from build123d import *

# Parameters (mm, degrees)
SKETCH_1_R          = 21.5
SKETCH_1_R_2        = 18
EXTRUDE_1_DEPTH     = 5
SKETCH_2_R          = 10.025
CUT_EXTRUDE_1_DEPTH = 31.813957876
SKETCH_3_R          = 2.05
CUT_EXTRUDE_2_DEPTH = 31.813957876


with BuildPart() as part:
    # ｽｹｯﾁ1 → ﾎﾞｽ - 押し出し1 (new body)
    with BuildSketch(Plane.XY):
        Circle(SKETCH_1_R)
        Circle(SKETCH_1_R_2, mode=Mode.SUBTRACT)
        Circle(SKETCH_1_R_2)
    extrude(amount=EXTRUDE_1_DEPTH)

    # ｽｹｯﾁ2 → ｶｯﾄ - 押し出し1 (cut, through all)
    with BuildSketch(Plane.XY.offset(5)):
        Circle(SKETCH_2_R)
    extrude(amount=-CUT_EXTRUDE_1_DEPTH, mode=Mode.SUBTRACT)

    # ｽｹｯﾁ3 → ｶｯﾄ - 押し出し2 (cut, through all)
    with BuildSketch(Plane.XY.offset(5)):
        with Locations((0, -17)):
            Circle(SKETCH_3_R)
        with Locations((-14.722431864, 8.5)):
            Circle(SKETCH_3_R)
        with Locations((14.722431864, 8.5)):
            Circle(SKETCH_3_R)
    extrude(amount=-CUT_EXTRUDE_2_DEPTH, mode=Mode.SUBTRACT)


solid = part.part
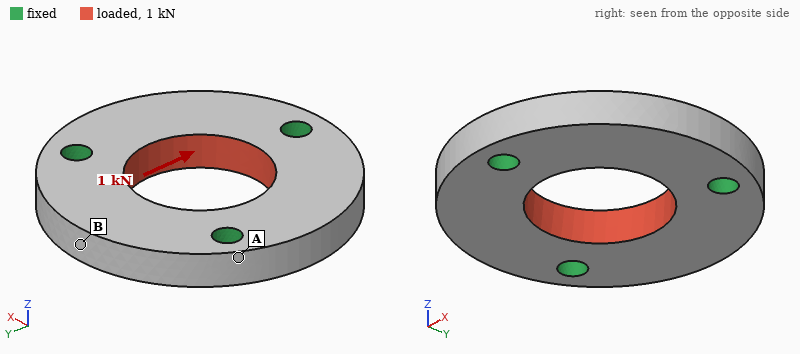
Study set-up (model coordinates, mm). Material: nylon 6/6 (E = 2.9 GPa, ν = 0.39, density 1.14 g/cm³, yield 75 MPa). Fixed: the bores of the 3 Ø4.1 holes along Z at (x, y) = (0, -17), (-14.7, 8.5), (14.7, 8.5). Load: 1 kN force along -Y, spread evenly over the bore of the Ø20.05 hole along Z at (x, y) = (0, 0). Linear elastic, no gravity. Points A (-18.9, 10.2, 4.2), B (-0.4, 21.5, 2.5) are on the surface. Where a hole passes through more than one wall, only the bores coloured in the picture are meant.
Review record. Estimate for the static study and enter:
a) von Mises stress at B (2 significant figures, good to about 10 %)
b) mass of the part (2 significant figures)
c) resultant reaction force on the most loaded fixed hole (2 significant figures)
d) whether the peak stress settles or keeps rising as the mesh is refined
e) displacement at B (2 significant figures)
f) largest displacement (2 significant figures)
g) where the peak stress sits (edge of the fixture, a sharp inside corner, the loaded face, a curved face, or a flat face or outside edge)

4.7 MPa
6.3 g
370 N
keeps rising
32 µm
42 µm
edge of the fixture
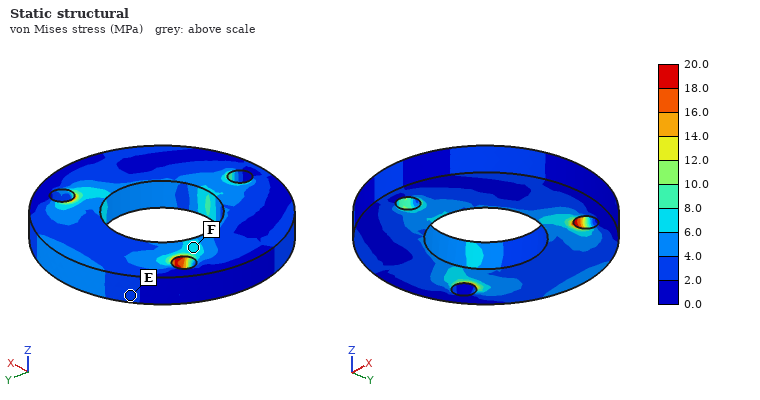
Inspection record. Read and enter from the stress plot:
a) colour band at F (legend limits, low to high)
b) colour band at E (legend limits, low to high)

6.0 to 8.0 MPa
2.0 to 4.0 MPa
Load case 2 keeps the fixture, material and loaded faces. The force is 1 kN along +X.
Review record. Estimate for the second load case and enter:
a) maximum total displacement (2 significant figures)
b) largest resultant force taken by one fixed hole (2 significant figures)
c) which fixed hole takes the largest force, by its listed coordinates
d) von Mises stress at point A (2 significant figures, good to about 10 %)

38 µm
400 N
(0, -17)
3.0 MPa
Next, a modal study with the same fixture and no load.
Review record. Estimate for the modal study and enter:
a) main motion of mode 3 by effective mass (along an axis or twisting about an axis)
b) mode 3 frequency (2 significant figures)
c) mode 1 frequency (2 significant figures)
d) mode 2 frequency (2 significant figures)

along Z
6000 Hz
5600 Hz
5600 Hz
